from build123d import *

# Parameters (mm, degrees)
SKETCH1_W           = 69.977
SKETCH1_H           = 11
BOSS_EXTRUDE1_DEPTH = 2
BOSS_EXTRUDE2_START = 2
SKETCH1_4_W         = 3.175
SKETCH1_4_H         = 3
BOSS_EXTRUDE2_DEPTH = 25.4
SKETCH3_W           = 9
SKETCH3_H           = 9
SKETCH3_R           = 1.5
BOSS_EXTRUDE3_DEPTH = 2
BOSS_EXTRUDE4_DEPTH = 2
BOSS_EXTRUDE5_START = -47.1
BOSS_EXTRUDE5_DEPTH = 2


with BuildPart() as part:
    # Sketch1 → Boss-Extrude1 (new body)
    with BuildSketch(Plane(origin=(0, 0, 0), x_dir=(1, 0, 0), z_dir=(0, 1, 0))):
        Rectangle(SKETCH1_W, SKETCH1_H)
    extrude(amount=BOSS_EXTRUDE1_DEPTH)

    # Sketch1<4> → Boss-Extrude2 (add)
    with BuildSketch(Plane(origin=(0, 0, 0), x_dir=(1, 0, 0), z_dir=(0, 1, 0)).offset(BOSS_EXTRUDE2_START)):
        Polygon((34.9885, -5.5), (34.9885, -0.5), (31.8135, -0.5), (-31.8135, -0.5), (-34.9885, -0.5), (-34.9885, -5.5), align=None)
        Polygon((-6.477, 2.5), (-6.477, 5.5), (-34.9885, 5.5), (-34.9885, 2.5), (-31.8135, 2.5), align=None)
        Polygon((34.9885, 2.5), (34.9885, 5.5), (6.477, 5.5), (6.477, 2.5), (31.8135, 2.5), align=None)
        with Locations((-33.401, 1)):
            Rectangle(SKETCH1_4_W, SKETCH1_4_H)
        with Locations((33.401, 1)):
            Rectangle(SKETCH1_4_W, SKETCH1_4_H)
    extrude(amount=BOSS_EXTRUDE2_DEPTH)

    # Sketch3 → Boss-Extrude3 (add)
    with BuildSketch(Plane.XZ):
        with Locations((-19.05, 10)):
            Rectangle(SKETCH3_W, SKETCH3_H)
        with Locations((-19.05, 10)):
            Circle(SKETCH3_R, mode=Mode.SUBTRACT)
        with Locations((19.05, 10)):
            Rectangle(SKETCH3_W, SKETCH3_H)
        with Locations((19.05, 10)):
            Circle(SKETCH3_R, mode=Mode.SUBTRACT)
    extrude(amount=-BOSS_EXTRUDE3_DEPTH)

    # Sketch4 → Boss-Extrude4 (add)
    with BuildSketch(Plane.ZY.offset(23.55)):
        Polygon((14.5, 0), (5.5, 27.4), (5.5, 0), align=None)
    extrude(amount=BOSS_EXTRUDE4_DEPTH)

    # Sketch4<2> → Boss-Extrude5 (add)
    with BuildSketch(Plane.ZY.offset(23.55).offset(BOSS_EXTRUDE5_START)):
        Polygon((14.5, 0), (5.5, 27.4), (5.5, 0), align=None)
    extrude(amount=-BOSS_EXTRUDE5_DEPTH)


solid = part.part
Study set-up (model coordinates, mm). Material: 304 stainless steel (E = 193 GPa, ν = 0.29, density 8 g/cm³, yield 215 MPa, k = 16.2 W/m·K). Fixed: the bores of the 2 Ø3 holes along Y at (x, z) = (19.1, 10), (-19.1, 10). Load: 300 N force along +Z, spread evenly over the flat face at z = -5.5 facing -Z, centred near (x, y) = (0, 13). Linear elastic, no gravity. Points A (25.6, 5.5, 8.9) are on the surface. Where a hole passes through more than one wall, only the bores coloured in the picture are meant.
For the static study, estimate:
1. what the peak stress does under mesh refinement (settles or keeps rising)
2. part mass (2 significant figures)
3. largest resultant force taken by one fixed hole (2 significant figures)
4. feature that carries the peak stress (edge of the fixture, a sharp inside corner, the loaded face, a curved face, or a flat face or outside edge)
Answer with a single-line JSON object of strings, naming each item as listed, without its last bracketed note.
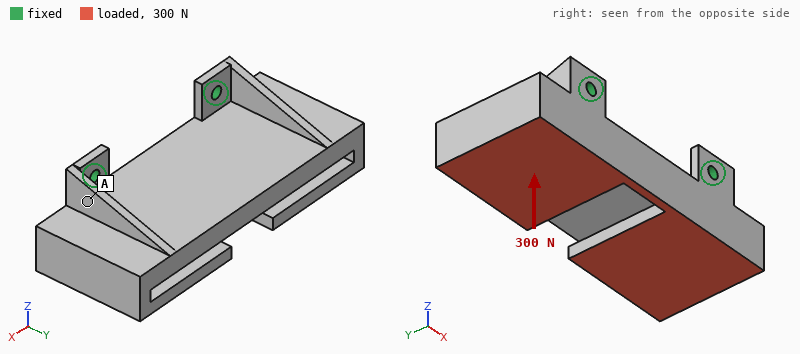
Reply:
{"what the peak stress does under mesh refinement": "keeps rising", "part mass": "130 g", "largest resultant force taken by one fixed hole": "150 N", "feature that carries the peak stress": "edge of the fixture"}
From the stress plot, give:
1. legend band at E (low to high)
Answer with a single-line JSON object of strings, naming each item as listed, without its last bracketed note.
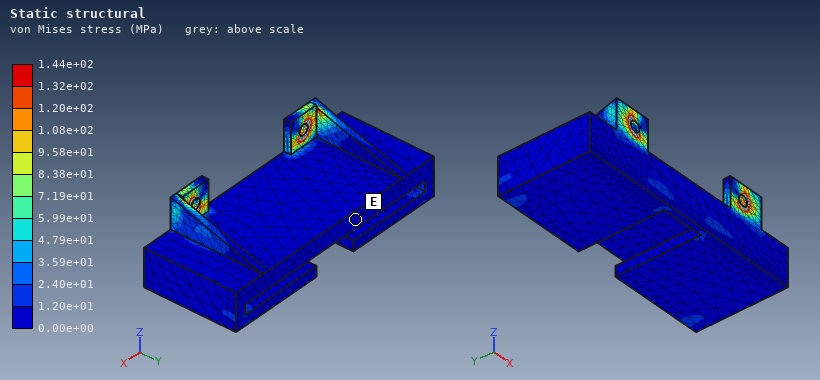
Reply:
{"legend band at E": "0.00e+00 to 1.20e+01 MPa"}
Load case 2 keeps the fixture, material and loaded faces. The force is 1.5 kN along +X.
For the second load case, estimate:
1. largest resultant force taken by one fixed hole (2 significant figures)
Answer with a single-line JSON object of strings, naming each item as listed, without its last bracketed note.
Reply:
{"largest resultant force taken by one fixed hole": "1000 N"}
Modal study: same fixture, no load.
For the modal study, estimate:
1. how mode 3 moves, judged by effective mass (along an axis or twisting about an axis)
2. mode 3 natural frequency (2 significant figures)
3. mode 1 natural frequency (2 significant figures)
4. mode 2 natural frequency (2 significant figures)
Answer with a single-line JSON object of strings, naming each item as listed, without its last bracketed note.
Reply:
{"how mode 3 moves, judged by effective mass": "along X", "mode 3 natural frequency": "4800 Hz", "mode 1 natural frequency": "1000 Hz", "mode 2 natural frequency": "2700 Hz"}
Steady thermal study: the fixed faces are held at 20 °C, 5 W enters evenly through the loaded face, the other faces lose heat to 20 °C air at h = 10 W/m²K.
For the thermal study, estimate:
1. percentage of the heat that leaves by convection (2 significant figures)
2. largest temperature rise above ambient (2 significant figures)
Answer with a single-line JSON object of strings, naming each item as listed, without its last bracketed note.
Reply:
{"percentage of the heat that leaves by convection": "41 %", "largest temperature rise above ambient": "41 K"}
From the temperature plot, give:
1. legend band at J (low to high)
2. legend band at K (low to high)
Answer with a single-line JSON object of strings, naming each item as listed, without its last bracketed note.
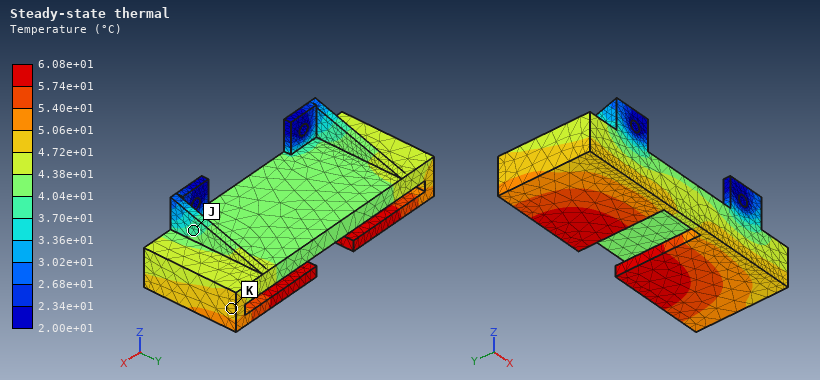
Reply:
{"legend band at J": "3.70e+01 to 4.04e+01 °C", "legend band at K": "4.72e+01 to 5.06e+01 °C"}
